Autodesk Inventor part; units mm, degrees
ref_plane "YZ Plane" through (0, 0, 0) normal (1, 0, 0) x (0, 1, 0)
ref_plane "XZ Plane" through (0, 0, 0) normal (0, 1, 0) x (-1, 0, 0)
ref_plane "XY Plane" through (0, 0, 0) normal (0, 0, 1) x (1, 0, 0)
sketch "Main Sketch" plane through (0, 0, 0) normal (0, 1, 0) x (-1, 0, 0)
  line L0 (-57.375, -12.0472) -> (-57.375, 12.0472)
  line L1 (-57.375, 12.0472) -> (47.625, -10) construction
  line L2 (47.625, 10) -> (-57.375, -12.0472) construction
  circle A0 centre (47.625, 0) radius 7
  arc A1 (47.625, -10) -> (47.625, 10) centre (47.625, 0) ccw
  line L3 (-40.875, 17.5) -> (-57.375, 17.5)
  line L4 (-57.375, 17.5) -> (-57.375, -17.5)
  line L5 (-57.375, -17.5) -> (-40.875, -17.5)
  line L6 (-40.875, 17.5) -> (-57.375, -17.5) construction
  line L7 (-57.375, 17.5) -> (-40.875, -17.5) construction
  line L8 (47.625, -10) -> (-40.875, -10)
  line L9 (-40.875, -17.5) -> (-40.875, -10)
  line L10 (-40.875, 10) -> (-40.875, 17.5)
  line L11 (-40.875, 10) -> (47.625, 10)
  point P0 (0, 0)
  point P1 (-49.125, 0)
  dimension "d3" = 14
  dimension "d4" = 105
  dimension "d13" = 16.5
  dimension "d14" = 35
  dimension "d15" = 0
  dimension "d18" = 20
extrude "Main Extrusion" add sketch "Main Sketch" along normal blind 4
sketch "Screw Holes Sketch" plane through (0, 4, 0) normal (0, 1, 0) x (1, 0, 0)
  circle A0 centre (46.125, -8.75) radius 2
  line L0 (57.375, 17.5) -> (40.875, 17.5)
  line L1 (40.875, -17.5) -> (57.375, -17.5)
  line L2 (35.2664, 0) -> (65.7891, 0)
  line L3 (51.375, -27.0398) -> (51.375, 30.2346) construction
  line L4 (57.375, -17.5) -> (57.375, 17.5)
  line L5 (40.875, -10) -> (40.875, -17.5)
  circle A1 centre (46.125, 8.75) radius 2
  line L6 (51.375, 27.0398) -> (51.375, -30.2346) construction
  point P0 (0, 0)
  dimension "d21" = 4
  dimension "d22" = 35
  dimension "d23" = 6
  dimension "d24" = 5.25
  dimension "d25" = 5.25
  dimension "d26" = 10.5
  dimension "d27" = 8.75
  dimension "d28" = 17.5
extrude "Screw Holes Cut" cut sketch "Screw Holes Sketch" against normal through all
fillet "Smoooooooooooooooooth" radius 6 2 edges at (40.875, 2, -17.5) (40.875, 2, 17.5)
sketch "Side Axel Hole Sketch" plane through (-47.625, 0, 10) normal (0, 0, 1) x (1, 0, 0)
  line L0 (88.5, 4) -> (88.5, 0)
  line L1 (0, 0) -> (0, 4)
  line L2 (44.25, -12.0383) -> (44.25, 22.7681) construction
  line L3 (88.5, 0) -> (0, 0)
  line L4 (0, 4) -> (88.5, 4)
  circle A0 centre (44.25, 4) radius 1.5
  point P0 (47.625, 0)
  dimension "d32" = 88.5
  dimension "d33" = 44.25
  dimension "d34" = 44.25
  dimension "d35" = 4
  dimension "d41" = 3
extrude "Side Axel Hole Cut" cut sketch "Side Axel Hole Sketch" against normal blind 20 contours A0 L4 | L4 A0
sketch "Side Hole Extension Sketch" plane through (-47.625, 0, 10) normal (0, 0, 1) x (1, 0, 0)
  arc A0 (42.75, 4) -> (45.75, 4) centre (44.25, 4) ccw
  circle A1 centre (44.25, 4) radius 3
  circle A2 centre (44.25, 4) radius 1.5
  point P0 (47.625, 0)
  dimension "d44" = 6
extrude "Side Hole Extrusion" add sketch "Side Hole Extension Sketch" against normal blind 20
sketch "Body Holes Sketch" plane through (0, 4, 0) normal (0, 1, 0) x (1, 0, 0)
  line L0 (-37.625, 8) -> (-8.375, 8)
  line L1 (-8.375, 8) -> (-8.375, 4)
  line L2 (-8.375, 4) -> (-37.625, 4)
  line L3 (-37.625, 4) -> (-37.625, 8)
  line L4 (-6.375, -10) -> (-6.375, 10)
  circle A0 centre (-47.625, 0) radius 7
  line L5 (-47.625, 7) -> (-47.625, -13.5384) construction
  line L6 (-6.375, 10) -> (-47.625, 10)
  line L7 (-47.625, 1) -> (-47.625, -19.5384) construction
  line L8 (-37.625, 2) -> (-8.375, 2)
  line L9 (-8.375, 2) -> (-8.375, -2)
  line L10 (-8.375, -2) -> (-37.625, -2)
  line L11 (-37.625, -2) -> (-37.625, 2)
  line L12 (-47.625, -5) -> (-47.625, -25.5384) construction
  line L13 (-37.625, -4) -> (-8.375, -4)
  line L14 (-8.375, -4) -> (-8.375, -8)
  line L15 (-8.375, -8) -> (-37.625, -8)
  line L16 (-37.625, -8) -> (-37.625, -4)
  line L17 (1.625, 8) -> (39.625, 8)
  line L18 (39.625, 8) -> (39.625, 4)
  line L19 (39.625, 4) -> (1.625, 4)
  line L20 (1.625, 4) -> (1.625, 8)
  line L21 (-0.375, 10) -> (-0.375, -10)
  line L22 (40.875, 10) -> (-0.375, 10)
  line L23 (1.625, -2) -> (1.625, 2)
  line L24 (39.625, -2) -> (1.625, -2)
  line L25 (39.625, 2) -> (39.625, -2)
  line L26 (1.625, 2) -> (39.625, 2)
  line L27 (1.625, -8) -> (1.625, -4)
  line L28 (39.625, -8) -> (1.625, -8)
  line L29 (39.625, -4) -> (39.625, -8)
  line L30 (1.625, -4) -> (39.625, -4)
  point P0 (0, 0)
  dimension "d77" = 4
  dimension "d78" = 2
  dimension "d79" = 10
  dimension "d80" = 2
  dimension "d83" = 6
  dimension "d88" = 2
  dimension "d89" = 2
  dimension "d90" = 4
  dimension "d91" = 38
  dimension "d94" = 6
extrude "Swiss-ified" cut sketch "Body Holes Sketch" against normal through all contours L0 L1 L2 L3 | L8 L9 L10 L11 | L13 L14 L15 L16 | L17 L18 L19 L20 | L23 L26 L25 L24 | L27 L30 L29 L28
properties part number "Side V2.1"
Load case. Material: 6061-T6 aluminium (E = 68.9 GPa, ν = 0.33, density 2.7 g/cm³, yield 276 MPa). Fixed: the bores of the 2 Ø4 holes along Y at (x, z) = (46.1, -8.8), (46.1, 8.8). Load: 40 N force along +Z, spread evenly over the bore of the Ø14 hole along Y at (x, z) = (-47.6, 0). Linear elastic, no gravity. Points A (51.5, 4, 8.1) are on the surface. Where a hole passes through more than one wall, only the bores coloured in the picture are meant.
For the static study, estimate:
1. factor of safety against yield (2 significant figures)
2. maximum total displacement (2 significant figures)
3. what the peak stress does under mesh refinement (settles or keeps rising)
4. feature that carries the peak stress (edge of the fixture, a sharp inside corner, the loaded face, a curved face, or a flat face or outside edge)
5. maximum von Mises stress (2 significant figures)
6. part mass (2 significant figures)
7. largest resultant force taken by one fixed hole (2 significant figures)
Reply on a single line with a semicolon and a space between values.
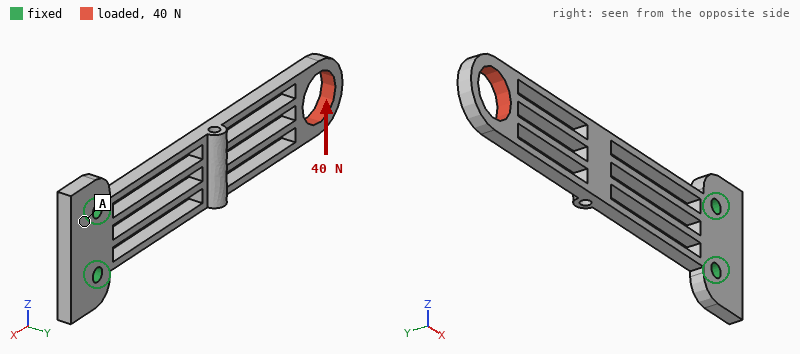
3.4; 0.52 mm; settles; a flat face or outside edge; 81 MPa; 17 g; 210 N
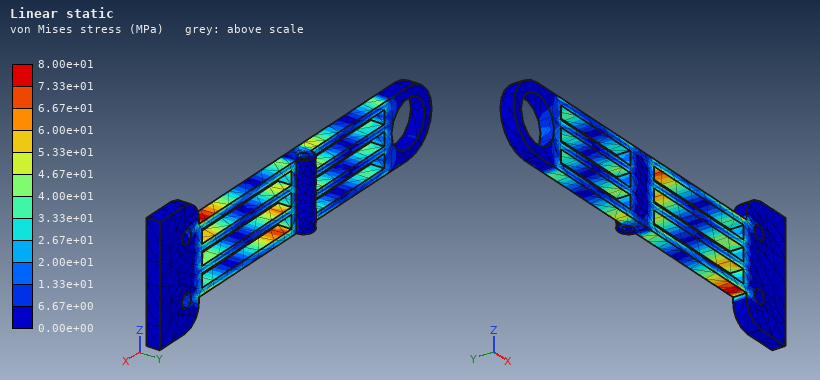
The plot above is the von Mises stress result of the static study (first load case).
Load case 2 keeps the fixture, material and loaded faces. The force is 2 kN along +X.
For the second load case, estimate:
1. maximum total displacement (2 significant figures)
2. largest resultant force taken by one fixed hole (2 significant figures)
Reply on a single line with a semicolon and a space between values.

0.11 mm; 1.0 kN
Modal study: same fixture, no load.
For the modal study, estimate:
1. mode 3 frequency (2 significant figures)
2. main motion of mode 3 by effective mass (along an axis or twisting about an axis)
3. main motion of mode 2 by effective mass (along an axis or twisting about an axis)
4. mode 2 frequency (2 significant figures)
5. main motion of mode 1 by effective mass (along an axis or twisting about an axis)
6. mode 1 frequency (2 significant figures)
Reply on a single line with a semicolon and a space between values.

1500 Hz; twisting about X; along Z; 600 Hz; along Y; 300 Hz
